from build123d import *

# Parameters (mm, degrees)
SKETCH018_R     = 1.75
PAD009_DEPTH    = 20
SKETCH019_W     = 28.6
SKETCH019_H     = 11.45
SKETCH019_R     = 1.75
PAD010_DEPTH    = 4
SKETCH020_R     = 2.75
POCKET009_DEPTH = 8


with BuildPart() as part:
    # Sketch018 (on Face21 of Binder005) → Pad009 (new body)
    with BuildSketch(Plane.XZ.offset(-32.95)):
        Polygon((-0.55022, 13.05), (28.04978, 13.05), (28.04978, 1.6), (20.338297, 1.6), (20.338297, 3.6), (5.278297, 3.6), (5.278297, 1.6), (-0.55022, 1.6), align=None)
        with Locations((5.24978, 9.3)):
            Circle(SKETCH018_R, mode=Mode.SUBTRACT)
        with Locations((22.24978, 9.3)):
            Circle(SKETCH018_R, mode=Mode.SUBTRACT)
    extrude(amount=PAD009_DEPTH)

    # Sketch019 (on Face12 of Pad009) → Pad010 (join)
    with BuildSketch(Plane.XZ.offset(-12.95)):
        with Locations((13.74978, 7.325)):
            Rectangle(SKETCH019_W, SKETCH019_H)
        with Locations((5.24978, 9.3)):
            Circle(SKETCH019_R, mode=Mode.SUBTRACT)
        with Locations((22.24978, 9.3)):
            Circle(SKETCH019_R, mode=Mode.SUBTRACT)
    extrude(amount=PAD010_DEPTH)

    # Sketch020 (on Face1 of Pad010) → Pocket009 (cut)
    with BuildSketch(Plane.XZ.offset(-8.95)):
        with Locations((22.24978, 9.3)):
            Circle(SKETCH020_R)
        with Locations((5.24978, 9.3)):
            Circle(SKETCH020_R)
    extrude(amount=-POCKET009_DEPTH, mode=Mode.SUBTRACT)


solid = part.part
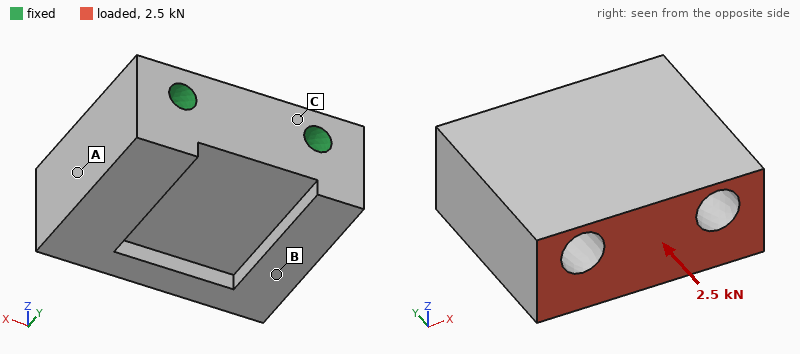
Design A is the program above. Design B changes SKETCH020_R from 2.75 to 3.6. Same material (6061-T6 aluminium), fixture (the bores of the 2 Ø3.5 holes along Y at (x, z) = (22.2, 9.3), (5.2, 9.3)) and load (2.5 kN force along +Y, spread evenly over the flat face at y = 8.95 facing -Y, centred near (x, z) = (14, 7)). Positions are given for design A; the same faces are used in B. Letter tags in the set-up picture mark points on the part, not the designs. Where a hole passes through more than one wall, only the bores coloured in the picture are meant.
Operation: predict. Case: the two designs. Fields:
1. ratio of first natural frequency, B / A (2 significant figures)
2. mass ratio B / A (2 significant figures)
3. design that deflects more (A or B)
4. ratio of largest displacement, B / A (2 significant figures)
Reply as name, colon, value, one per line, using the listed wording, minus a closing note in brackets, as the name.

ratio of first natural frequency, B / A: 0.98
mass ratio B / A: 0.96
design that deflects more: B
ratio of largest displacement, B / A: 1.2
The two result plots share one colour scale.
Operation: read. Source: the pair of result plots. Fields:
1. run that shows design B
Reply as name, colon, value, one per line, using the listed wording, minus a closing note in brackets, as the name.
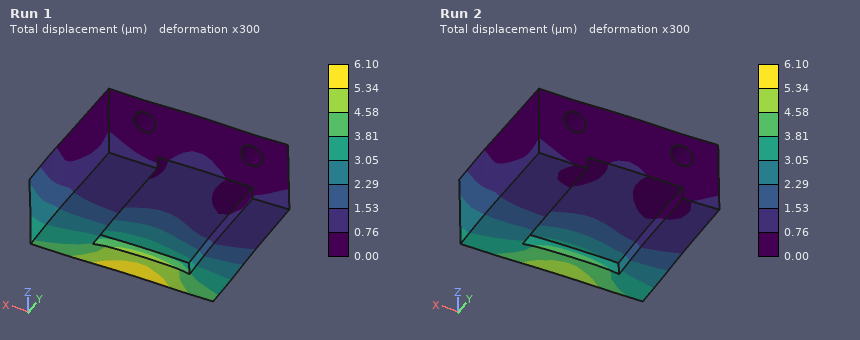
run that shows design B: Run 1
